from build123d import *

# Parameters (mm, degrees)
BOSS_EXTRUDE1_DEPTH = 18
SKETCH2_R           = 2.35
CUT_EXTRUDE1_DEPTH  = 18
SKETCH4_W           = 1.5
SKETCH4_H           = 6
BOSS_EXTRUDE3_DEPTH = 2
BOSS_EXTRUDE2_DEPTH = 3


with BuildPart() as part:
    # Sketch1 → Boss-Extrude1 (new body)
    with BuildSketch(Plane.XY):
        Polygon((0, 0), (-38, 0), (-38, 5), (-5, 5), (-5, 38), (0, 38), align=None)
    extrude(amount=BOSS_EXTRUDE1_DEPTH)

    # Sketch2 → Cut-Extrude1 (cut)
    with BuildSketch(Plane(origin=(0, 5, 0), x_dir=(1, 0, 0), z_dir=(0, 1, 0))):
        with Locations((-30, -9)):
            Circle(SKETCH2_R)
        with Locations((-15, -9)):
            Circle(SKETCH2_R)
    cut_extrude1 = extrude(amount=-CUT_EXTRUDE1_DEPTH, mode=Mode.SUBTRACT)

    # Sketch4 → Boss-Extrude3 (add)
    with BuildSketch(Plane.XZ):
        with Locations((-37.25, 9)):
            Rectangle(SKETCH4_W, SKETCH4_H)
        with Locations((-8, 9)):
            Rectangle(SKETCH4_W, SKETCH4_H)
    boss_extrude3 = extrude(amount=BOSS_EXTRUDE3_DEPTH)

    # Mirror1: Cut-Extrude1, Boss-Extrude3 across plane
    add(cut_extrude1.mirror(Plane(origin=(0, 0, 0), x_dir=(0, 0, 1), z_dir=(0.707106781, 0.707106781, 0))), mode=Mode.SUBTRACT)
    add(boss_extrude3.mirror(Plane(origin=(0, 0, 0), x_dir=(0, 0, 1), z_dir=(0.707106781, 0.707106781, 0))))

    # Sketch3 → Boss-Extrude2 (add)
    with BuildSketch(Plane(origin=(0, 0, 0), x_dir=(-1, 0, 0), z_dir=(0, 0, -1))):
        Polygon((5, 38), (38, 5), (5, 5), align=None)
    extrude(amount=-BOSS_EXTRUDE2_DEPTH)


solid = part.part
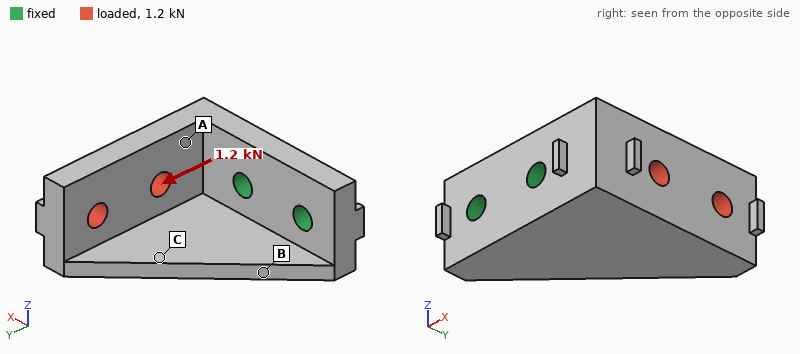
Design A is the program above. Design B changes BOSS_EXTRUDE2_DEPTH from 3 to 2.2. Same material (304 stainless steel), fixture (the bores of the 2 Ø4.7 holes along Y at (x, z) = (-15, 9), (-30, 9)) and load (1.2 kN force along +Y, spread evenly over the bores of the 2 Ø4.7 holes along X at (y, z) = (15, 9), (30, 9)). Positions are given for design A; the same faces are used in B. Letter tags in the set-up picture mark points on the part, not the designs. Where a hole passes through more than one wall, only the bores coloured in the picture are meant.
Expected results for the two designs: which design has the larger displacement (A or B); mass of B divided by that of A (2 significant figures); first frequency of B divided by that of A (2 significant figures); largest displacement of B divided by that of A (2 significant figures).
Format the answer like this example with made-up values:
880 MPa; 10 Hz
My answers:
B; 0.94; 0.98; 1.2
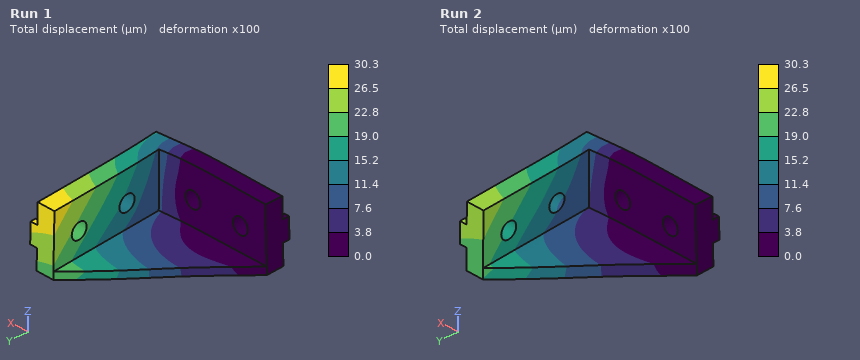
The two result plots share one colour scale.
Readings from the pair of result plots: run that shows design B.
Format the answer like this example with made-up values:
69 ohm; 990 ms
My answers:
Run 1
